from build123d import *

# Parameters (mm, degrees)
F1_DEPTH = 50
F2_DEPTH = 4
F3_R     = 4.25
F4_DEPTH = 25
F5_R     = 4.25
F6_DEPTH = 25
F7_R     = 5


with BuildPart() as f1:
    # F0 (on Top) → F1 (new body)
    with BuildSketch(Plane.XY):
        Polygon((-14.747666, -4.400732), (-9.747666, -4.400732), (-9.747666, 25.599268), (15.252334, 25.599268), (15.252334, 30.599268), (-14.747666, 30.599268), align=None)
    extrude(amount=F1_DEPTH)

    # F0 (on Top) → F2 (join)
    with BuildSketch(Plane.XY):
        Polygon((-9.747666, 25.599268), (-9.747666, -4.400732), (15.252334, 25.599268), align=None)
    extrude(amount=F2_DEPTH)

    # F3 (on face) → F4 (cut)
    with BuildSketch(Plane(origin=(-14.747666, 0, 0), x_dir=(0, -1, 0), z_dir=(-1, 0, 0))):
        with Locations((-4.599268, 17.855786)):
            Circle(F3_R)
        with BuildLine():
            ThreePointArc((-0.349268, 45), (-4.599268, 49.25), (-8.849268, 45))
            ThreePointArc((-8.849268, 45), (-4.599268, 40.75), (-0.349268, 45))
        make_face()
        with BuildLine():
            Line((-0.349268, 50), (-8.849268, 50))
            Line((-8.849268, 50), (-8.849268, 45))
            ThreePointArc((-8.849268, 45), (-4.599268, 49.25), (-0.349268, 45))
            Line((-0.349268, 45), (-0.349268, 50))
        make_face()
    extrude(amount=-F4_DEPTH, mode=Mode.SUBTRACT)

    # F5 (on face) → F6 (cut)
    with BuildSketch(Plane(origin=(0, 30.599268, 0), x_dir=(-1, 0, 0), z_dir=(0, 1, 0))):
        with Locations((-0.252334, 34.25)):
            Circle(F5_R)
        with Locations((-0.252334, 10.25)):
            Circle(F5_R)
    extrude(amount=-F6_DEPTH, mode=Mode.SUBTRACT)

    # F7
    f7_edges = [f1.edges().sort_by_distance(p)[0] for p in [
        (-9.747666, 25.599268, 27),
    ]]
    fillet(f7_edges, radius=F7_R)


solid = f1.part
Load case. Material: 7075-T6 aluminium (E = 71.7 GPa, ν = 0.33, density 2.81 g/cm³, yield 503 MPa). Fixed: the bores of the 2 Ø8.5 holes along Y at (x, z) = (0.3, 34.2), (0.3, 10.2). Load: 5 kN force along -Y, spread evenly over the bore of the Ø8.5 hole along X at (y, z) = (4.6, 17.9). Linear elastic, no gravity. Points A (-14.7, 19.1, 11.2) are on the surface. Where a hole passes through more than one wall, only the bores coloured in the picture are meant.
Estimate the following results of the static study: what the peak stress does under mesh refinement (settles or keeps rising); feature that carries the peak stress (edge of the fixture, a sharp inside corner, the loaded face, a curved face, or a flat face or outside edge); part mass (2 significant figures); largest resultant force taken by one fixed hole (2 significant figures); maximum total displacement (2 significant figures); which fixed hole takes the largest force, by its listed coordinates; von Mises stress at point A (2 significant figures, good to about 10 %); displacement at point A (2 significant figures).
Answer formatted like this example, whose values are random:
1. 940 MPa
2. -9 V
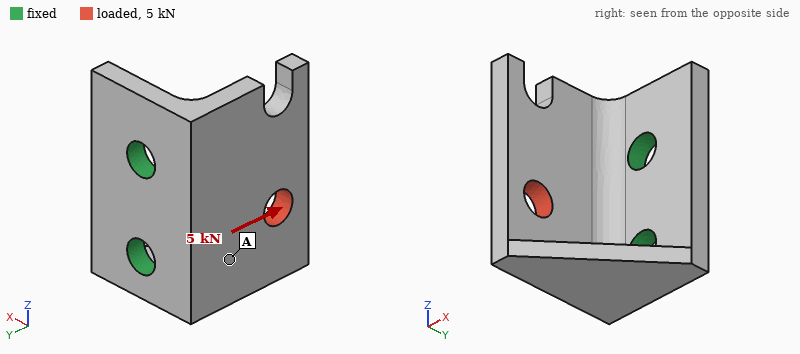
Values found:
1. keeps rising
2. edge of the fixture
3. 44 g
4. 3.2 kN
5. 0.16 mm
6. (0.3, 10.2)
7. 43 MPa
8. 0.072 mm
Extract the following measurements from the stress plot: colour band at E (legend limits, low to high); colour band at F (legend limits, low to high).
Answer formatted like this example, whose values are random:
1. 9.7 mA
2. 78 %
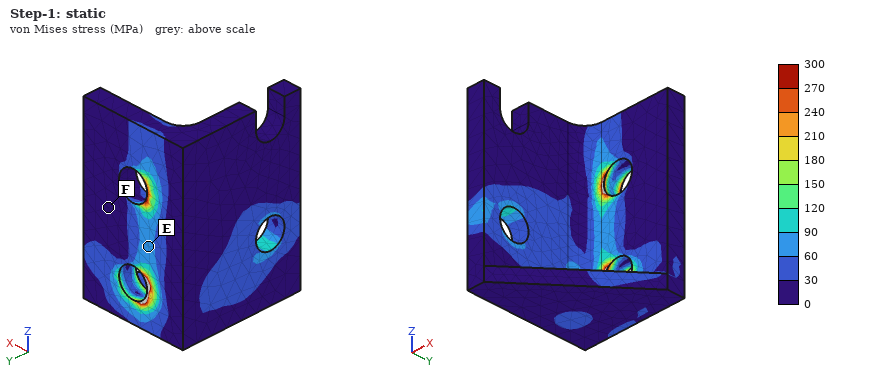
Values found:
1. 60 to 90 MPa
2. 0 to 30 MPa
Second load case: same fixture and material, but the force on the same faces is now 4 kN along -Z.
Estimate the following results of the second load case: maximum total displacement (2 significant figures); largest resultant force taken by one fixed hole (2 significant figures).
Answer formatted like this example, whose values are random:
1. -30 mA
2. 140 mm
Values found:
1. 0.16 mm
2. 3.9 kN
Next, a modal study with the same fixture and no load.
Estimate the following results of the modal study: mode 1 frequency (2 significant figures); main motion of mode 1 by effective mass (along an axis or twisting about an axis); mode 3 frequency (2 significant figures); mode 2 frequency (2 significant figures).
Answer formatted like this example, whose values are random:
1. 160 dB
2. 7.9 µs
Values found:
1. 4100 Hz
2. along X
3. 9900 Hz
4. 6500 Hz
